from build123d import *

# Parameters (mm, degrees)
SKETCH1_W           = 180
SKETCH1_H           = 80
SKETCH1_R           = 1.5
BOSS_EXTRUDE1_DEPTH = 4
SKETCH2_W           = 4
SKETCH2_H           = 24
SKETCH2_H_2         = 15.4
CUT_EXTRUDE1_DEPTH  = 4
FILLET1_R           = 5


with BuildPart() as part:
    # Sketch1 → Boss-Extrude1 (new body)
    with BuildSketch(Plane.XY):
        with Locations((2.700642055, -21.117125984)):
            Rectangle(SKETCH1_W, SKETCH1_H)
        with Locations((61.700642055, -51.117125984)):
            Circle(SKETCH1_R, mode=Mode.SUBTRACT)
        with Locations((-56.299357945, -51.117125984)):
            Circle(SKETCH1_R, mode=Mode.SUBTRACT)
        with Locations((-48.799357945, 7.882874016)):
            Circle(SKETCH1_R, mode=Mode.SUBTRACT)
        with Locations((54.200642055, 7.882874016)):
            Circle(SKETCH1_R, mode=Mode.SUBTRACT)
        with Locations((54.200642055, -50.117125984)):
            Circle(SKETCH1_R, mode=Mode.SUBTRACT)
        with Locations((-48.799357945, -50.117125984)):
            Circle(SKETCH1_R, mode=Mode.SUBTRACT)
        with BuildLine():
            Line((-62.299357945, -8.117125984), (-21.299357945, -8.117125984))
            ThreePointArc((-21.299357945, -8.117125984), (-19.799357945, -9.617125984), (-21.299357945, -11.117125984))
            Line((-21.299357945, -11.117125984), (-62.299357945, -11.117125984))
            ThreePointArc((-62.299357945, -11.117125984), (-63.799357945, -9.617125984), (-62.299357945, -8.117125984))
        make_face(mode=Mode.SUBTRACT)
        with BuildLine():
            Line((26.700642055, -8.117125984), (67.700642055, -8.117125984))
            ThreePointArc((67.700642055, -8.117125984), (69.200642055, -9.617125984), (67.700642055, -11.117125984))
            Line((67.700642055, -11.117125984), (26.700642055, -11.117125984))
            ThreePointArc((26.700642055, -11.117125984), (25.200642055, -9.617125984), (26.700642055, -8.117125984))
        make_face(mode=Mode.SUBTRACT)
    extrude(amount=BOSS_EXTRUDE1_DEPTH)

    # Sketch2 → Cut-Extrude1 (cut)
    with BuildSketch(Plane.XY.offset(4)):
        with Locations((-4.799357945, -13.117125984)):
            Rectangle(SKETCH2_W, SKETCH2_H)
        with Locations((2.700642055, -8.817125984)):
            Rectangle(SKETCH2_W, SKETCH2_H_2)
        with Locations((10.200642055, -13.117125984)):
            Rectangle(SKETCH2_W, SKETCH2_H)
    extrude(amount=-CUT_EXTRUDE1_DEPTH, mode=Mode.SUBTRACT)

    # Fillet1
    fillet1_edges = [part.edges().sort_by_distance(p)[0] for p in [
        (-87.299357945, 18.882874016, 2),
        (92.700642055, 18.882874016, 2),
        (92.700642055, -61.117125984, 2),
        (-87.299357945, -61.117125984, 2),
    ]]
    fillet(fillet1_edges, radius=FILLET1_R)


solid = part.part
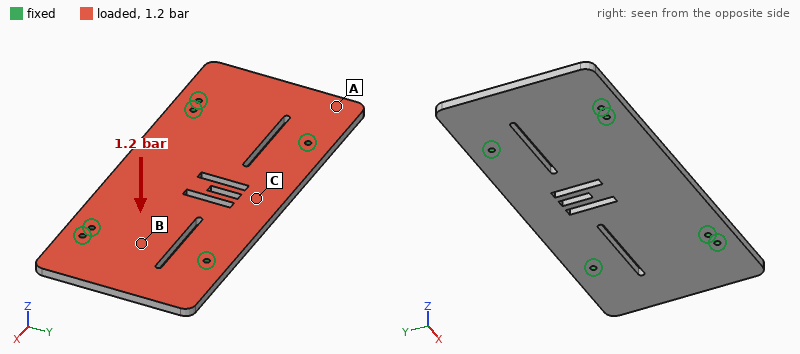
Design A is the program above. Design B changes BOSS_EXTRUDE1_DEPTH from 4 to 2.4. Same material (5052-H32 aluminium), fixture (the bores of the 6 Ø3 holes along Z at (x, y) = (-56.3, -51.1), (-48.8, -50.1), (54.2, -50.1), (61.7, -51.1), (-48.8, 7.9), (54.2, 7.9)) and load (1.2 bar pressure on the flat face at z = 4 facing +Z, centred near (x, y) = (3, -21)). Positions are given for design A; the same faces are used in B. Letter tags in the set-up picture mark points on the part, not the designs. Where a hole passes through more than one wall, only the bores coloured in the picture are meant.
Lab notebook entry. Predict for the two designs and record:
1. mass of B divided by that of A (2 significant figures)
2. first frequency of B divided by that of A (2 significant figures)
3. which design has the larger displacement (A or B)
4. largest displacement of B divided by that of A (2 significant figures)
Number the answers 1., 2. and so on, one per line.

1. 0.60
2. 0.62
3. B
4. 4.4
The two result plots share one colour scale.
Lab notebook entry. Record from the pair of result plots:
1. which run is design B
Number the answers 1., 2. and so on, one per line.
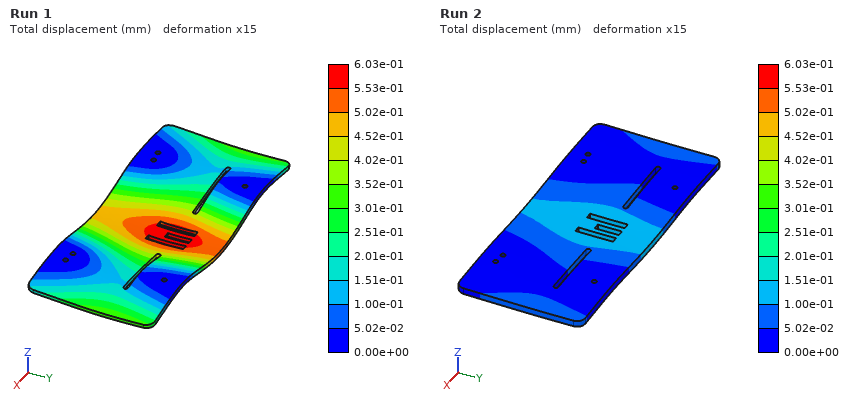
1. Run 1
